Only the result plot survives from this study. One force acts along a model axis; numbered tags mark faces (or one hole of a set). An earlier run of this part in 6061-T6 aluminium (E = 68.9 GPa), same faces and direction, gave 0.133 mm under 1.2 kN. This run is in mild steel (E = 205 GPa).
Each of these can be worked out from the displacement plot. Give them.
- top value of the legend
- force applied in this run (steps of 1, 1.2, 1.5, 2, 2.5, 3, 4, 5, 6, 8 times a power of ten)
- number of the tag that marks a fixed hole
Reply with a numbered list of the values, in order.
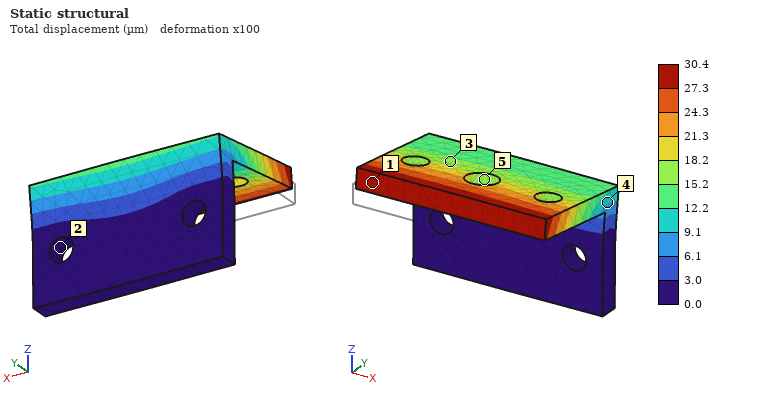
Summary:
1. 30.4 µm
2. 800 N
3. 2
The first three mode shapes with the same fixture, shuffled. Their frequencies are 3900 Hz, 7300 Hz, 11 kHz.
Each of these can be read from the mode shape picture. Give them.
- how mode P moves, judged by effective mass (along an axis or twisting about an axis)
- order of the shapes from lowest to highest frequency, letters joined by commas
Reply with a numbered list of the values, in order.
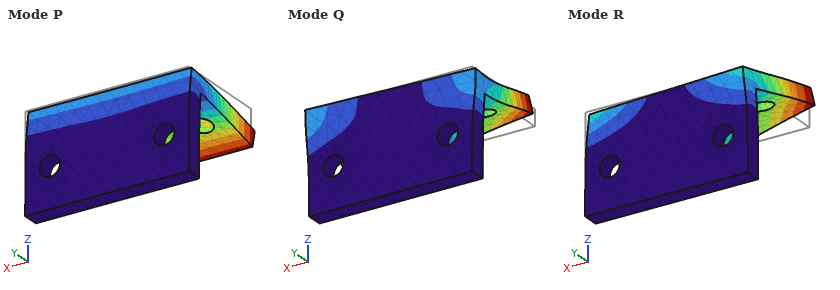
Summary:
1. along Z
2. P, R, Q
